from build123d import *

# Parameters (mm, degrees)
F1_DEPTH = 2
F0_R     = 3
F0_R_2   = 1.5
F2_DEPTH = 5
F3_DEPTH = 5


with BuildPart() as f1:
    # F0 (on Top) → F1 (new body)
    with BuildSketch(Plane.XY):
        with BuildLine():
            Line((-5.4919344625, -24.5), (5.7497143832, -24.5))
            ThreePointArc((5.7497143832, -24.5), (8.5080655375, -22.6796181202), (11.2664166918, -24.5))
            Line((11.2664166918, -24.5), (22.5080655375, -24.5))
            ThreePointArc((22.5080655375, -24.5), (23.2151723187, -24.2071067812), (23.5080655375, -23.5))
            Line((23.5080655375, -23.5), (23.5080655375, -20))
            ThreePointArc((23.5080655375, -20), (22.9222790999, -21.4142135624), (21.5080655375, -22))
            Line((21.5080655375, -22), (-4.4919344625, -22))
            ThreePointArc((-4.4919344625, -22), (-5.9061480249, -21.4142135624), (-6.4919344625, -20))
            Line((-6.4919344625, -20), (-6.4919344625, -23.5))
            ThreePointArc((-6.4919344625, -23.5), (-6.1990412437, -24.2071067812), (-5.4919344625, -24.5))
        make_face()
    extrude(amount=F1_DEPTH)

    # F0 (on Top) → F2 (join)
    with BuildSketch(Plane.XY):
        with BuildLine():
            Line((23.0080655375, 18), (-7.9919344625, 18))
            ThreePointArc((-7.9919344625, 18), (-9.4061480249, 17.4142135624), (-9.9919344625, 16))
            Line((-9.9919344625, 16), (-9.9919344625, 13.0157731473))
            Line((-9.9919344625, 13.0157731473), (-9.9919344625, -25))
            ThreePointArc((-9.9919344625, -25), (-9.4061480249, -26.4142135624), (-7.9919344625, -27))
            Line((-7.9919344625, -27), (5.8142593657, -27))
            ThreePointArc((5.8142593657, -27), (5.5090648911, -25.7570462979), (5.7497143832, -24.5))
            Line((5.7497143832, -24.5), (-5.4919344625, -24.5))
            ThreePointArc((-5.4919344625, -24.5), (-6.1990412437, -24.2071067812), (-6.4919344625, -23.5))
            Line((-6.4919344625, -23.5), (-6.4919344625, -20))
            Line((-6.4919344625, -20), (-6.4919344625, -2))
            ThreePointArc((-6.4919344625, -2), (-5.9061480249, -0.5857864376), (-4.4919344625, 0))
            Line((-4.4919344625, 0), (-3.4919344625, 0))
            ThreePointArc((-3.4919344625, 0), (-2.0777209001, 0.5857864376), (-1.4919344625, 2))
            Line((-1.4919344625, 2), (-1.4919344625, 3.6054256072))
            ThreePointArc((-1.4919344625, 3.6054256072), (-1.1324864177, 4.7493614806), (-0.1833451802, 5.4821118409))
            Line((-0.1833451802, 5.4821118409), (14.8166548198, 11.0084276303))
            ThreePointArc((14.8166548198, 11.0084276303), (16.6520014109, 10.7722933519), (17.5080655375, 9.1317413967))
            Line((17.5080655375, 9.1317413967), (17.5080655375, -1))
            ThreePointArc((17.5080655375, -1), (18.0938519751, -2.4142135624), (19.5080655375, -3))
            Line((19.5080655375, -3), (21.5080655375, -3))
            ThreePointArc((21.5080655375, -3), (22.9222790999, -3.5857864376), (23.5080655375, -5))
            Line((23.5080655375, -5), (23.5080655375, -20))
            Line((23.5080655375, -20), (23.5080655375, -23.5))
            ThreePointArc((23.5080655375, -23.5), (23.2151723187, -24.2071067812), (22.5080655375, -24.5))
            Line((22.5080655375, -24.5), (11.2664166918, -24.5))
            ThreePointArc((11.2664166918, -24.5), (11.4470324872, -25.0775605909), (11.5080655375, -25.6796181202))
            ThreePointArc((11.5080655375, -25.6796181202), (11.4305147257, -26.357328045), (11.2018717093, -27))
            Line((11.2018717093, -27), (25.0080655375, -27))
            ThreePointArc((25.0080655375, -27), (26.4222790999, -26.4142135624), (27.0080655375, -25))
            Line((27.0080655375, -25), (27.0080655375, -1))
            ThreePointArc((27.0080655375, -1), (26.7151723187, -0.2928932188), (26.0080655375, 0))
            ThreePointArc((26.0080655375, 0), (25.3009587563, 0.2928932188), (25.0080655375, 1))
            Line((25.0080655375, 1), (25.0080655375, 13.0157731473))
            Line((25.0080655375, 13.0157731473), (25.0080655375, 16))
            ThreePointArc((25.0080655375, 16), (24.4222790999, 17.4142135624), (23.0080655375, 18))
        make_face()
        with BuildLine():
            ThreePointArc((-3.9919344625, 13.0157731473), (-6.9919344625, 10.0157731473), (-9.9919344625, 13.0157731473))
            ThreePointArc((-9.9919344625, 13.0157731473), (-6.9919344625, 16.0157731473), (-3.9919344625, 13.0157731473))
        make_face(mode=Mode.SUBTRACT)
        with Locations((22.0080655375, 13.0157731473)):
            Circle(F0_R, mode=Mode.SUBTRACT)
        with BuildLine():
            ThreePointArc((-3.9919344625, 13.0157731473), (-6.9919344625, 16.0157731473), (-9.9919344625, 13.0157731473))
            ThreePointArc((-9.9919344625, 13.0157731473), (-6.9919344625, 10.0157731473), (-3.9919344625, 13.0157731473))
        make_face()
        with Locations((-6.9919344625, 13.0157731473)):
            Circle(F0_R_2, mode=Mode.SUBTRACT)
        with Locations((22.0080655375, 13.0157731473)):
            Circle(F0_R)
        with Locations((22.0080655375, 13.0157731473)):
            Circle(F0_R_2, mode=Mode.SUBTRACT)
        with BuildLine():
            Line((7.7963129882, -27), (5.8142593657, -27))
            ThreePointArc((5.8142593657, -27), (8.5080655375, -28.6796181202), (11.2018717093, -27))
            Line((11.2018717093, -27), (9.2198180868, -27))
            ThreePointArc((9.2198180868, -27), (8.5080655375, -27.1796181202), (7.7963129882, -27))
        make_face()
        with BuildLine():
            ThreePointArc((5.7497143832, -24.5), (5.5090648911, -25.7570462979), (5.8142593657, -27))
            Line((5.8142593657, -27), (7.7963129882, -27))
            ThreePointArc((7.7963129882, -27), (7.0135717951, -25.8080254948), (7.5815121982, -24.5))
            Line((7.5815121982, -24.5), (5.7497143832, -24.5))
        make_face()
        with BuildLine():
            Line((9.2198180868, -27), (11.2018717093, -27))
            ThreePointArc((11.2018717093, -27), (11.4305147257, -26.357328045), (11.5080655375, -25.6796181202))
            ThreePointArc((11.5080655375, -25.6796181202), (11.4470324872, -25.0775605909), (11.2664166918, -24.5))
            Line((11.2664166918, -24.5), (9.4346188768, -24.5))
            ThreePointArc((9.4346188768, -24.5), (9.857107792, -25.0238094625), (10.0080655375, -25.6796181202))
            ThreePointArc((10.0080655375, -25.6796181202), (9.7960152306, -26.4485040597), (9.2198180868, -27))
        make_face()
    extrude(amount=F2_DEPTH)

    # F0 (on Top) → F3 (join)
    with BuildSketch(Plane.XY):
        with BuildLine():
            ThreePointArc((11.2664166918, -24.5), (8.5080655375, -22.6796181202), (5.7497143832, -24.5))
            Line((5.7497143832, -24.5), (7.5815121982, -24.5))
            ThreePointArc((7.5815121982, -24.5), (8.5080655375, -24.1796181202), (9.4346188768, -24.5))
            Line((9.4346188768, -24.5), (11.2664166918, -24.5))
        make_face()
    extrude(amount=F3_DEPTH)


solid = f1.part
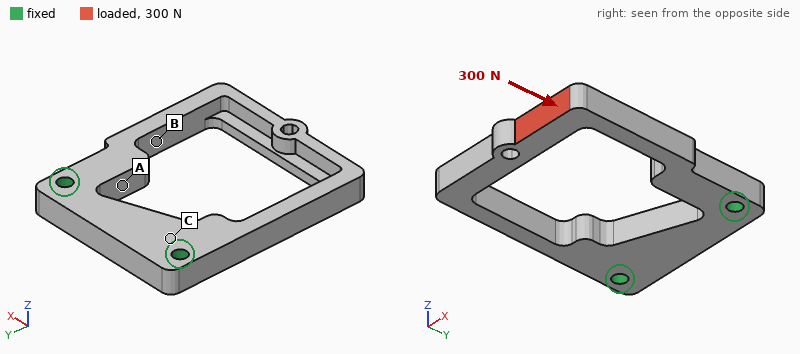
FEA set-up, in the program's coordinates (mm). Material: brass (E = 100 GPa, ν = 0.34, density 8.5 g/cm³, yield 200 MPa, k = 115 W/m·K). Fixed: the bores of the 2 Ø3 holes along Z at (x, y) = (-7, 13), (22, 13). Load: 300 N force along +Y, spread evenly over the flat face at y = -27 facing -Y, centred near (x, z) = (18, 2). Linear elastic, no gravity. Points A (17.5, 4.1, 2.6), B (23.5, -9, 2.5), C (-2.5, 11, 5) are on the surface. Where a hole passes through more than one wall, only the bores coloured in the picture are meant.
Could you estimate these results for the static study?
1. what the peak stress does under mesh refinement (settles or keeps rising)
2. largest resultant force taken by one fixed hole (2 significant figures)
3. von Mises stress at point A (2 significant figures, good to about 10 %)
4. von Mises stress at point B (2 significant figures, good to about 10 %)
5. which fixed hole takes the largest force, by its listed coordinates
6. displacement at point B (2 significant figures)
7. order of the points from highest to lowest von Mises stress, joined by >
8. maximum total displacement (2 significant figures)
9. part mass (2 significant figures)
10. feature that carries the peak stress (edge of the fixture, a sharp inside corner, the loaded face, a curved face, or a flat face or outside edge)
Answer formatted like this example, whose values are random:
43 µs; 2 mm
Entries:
keeps rising; 240 N; 15 MPa; 36 MPa; (22, 13); 15 µm; B > A > C; 36 µm; 33 g; a sharp inside corner
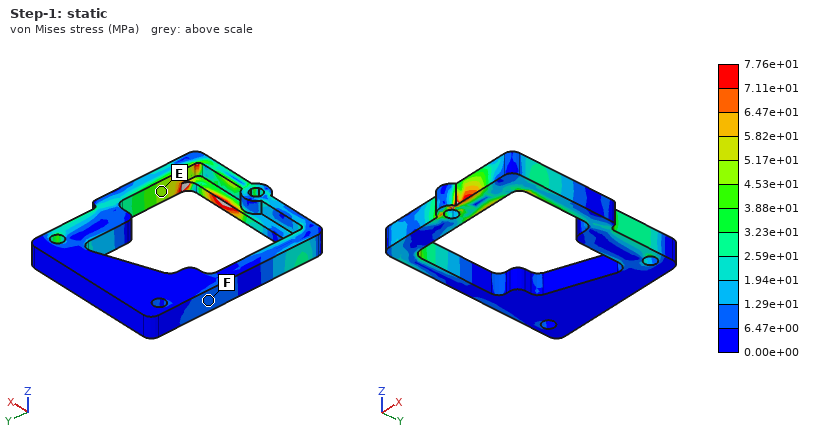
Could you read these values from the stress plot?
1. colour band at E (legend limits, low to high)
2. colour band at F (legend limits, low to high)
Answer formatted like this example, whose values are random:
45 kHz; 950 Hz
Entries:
4.53e+01 to 5.17e+01 MPa; 6.47e+00 to 1.29e+01 MPa
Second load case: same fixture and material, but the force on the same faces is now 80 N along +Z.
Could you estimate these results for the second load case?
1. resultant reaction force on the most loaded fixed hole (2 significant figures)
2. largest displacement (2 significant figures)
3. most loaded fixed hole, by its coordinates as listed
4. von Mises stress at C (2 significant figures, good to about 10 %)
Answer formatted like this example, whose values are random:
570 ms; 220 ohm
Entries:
61 N; 0.19 mm; (22, 13); 12 MPa
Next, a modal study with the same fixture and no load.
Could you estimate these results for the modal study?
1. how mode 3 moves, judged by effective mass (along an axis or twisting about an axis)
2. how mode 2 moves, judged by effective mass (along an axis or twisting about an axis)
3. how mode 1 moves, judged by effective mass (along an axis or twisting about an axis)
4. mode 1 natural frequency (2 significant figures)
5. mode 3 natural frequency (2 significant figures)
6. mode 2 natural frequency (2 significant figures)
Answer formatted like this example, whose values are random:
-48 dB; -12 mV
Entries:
twisting about Y; along X; along Z; 1400 Hz; 2700 Hz; 2300 Hz
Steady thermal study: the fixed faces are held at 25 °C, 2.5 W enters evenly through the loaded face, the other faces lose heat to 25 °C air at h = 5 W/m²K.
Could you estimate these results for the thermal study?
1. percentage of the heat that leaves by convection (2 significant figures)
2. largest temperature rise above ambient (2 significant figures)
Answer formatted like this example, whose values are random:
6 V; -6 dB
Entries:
4.7 %; 25 K
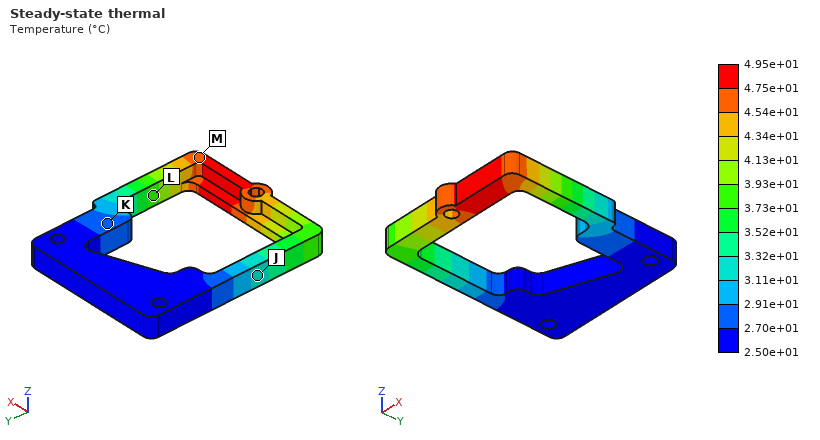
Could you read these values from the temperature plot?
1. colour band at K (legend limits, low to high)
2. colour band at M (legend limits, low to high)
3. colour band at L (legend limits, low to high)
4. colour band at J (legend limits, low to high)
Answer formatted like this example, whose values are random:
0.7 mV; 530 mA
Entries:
2.70e+01 to 2.91e+01 °C; 4.54e+01 to 4.75e+01 °C; 3.73e+01 to 3.93e+01 °C; 3.11e+01 to 3.32e+01 °C
